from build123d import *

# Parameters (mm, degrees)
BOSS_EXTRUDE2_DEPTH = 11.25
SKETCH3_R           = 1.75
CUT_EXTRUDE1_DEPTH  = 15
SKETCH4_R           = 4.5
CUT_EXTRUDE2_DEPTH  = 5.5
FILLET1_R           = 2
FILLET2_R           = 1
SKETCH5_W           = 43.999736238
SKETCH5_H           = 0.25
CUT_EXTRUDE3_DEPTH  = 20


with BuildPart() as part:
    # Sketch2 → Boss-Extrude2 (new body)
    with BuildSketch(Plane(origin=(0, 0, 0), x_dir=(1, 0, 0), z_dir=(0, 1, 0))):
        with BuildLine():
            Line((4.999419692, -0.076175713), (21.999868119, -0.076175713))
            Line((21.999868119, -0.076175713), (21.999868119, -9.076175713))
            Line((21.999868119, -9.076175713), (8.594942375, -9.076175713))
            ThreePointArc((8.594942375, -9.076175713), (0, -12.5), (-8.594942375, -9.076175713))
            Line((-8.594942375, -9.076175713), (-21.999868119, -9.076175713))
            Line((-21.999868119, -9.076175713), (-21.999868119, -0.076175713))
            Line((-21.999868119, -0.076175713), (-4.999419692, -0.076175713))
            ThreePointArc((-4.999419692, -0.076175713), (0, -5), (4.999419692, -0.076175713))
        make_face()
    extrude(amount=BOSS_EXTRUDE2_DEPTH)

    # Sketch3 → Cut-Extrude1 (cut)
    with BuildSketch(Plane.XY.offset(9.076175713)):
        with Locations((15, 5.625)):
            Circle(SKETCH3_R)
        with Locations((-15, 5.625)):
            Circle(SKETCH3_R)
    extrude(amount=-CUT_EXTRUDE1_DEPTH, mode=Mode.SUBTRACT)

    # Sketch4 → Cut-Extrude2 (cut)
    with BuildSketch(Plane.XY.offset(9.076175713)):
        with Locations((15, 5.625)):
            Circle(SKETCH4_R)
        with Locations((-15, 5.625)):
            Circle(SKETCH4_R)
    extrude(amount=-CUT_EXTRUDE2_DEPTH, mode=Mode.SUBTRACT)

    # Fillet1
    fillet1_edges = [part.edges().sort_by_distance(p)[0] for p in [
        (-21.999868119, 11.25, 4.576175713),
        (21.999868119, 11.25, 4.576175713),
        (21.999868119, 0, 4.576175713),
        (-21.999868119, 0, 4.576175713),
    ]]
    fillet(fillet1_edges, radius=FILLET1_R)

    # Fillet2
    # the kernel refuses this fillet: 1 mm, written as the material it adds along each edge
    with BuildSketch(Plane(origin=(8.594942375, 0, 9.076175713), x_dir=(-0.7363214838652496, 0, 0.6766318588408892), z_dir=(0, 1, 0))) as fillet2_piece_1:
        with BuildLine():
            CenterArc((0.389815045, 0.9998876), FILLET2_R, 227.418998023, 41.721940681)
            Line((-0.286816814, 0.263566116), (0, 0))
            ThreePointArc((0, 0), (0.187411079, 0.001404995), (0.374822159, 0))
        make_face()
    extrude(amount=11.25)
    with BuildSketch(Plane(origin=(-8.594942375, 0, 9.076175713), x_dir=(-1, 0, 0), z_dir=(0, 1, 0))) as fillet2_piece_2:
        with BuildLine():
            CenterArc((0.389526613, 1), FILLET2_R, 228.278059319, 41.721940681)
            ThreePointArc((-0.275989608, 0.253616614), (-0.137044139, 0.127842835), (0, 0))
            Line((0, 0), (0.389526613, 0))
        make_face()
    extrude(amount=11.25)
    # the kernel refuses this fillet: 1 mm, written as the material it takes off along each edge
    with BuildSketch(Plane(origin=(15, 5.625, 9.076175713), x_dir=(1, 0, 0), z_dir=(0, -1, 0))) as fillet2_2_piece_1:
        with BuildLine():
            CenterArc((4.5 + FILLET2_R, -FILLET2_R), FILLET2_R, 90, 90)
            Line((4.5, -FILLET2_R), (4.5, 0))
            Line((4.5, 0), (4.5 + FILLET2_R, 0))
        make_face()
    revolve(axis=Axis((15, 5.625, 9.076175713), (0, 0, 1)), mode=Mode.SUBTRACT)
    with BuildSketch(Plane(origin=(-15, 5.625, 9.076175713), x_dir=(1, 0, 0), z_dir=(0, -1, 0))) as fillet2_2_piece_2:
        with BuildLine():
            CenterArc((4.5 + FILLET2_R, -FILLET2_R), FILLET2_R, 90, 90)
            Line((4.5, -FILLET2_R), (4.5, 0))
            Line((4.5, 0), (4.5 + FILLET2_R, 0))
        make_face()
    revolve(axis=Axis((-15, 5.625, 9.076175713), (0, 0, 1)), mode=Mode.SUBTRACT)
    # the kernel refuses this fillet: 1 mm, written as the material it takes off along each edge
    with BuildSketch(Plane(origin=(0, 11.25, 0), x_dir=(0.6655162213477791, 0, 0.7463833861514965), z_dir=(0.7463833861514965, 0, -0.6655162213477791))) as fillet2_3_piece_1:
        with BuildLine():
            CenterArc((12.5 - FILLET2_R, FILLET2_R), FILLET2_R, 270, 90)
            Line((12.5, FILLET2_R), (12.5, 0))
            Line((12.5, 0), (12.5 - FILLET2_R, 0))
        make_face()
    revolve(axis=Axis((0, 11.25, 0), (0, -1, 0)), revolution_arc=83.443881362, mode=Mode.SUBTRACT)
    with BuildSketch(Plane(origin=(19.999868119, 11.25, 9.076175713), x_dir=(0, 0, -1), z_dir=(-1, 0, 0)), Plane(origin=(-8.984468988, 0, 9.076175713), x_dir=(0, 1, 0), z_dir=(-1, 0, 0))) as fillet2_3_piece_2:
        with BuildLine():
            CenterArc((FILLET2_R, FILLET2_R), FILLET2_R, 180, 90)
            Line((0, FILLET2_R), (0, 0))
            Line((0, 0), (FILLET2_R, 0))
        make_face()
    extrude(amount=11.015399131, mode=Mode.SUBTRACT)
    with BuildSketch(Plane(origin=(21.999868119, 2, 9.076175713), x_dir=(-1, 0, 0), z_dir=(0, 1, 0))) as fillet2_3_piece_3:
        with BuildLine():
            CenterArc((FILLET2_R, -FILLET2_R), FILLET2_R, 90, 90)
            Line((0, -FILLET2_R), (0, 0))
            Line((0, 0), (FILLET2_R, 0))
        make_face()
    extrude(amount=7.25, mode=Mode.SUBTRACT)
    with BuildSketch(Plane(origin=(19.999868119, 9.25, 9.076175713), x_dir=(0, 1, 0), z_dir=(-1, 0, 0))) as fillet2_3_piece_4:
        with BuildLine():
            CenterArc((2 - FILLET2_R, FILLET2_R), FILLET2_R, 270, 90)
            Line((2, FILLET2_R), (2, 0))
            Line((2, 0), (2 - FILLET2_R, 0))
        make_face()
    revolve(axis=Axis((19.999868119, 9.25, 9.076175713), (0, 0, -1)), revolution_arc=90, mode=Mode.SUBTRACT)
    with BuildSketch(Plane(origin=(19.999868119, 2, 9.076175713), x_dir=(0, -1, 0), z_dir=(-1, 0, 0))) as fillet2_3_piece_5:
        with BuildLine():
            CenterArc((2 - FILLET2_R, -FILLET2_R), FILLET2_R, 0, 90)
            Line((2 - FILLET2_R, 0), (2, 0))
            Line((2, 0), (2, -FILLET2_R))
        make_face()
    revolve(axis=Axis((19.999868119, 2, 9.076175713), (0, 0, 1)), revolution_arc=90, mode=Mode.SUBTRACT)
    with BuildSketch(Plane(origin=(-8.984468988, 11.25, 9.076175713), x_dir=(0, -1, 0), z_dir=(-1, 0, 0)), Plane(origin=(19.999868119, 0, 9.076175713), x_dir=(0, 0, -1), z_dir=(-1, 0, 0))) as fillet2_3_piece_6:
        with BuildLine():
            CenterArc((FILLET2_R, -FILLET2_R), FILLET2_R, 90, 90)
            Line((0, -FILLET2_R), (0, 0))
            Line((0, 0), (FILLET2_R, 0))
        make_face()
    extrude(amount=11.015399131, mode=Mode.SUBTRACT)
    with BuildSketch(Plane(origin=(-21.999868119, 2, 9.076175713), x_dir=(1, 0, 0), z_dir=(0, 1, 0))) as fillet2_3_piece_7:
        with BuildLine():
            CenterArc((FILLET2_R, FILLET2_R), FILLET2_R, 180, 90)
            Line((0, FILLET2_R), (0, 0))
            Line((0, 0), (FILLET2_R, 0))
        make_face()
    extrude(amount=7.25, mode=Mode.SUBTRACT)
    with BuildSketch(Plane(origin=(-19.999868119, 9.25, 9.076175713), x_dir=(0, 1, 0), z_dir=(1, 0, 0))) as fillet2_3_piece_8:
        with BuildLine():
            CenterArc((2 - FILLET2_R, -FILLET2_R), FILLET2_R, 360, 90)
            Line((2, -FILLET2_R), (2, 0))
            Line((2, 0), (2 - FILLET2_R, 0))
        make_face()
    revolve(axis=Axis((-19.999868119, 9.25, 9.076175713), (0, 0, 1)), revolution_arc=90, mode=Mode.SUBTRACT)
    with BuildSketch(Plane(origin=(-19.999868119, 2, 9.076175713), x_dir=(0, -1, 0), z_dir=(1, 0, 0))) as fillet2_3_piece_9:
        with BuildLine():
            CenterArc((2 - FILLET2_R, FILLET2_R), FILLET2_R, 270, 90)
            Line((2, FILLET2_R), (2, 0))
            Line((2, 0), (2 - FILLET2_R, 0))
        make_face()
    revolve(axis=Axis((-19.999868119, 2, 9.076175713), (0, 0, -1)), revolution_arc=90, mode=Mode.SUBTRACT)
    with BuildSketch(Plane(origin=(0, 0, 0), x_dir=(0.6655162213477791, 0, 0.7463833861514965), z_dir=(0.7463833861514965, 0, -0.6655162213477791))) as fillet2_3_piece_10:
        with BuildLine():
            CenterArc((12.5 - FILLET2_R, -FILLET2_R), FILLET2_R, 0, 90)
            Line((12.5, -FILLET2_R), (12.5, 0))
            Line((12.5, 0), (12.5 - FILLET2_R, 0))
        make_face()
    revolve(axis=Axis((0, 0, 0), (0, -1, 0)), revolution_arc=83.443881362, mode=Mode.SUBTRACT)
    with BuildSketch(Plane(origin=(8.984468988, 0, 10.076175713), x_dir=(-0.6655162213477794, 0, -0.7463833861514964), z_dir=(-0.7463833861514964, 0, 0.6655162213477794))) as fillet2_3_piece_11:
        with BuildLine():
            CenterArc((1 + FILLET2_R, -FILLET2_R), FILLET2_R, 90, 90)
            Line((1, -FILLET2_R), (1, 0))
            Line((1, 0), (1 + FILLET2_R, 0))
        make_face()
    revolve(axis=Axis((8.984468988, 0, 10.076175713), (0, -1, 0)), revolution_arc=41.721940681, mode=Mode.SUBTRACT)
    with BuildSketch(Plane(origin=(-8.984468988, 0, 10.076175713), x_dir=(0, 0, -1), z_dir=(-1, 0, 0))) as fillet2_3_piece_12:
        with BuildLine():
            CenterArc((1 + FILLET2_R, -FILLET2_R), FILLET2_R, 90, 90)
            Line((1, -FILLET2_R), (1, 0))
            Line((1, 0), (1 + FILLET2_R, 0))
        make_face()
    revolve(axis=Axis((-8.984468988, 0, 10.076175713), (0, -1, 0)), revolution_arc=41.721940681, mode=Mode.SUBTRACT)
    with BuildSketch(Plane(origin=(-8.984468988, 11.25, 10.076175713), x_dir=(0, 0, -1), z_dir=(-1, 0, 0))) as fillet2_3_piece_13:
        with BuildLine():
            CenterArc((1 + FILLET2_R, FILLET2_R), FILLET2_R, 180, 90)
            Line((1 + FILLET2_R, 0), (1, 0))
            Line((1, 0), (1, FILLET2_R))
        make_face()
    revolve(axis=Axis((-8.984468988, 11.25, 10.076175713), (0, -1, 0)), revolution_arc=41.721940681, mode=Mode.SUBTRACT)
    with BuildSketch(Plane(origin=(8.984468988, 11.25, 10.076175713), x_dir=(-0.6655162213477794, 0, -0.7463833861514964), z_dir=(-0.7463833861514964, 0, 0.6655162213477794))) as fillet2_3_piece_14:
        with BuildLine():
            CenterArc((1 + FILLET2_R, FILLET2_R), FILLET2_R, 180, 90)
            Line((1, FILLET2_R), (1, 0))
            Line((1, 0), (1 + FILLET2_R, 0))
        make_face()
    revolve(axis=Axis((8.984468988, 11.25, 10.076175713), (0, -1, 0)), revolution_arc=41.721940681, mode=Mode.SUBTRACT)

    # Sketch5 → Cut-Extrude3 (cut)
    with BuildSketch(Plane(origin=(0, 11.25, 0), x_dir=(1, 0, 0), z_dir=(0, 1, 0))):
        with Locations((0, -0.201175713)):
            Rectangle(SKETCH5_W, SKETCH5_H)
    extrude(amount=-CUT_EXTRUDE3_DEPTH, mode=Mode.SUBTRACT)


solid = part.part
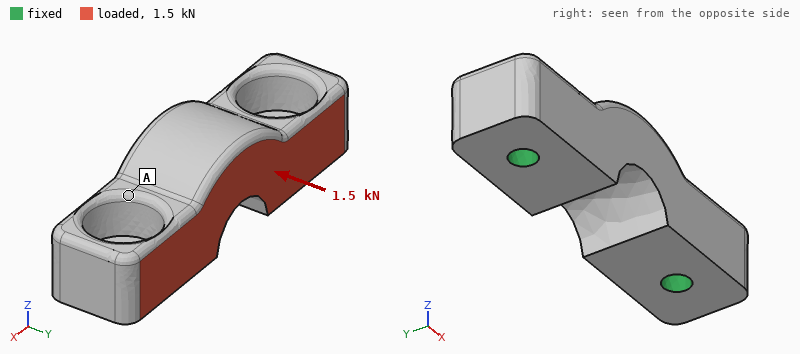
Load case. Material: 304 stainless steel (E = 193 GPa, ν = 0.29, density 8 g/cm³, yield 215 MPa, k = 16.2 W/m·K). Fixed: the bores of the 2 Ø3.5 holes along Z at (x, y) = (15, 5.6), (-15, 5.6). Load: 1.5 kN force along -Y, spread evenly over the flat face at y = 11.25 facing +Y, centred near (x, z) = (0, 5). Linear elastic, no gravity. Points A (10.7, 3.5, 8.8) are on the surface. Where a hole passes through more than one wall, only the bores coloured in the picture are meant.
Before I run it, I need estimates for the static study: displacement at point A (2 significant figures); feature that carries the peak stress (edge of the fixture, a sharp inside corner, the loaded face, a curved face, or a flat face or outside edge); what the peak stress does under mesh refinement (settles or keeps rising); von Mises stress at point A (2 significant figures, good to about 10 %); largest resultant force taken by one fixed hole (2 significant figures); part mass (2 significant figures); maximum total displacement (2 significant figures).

5.2 µm
edge of the fixture
keeps rising
21 MPa
750 N
28 g
9.0 µm
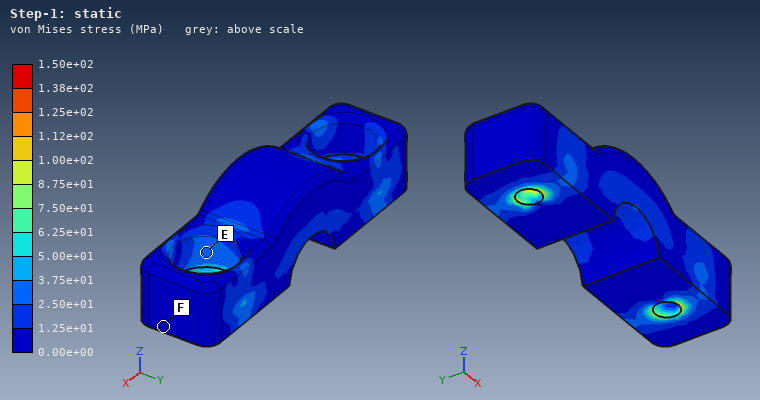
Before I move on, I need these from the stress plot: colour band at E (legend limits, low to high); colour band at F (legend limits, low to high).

2.50e+01 to 3.75e+01 MPa
0.00e+00 to 1.25e+01 MPa
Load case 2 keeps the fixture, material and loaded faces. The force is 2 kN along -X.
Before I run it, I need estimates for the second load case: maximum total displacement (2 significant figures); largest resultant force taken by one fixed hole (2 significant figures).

2.8 µm
1.1 kN
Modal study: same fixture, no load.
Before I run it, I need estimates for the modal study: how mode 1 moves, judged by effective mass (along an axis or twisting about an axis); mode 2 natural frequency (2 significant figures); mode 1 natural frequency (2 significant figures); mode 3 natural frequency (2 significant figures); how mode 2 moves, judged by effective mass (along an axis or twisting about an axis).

along Y
25 kHz
14 kHz
31 kHz
along Z
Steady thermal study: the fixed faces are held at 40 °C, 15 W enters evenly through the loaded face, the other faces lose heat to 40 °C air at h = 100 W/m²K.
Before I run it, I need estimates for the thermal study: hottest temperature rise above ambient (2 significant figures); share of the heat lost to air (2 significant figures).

48 K
29 %
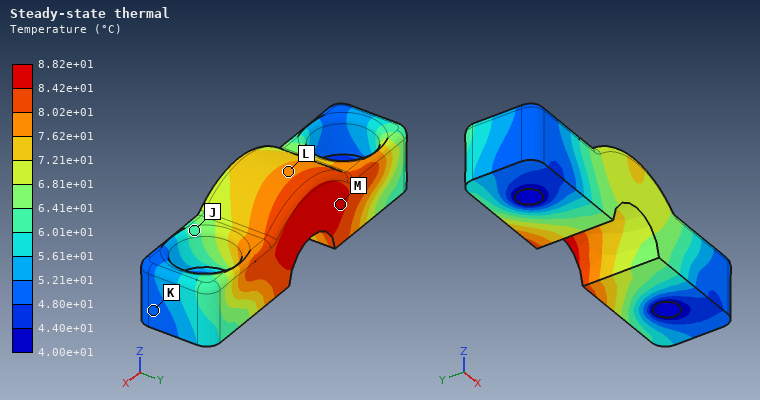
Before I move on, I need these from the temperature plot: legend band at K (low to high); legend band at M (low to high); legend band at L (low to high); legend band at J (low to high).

4.80e+01 to 5.21e+01 °C
8.42e+01 to 8.82e+01 °C
7.62e+01 to 8.02e+01 °C
6.01e+01 to 6.41e+01 °C
